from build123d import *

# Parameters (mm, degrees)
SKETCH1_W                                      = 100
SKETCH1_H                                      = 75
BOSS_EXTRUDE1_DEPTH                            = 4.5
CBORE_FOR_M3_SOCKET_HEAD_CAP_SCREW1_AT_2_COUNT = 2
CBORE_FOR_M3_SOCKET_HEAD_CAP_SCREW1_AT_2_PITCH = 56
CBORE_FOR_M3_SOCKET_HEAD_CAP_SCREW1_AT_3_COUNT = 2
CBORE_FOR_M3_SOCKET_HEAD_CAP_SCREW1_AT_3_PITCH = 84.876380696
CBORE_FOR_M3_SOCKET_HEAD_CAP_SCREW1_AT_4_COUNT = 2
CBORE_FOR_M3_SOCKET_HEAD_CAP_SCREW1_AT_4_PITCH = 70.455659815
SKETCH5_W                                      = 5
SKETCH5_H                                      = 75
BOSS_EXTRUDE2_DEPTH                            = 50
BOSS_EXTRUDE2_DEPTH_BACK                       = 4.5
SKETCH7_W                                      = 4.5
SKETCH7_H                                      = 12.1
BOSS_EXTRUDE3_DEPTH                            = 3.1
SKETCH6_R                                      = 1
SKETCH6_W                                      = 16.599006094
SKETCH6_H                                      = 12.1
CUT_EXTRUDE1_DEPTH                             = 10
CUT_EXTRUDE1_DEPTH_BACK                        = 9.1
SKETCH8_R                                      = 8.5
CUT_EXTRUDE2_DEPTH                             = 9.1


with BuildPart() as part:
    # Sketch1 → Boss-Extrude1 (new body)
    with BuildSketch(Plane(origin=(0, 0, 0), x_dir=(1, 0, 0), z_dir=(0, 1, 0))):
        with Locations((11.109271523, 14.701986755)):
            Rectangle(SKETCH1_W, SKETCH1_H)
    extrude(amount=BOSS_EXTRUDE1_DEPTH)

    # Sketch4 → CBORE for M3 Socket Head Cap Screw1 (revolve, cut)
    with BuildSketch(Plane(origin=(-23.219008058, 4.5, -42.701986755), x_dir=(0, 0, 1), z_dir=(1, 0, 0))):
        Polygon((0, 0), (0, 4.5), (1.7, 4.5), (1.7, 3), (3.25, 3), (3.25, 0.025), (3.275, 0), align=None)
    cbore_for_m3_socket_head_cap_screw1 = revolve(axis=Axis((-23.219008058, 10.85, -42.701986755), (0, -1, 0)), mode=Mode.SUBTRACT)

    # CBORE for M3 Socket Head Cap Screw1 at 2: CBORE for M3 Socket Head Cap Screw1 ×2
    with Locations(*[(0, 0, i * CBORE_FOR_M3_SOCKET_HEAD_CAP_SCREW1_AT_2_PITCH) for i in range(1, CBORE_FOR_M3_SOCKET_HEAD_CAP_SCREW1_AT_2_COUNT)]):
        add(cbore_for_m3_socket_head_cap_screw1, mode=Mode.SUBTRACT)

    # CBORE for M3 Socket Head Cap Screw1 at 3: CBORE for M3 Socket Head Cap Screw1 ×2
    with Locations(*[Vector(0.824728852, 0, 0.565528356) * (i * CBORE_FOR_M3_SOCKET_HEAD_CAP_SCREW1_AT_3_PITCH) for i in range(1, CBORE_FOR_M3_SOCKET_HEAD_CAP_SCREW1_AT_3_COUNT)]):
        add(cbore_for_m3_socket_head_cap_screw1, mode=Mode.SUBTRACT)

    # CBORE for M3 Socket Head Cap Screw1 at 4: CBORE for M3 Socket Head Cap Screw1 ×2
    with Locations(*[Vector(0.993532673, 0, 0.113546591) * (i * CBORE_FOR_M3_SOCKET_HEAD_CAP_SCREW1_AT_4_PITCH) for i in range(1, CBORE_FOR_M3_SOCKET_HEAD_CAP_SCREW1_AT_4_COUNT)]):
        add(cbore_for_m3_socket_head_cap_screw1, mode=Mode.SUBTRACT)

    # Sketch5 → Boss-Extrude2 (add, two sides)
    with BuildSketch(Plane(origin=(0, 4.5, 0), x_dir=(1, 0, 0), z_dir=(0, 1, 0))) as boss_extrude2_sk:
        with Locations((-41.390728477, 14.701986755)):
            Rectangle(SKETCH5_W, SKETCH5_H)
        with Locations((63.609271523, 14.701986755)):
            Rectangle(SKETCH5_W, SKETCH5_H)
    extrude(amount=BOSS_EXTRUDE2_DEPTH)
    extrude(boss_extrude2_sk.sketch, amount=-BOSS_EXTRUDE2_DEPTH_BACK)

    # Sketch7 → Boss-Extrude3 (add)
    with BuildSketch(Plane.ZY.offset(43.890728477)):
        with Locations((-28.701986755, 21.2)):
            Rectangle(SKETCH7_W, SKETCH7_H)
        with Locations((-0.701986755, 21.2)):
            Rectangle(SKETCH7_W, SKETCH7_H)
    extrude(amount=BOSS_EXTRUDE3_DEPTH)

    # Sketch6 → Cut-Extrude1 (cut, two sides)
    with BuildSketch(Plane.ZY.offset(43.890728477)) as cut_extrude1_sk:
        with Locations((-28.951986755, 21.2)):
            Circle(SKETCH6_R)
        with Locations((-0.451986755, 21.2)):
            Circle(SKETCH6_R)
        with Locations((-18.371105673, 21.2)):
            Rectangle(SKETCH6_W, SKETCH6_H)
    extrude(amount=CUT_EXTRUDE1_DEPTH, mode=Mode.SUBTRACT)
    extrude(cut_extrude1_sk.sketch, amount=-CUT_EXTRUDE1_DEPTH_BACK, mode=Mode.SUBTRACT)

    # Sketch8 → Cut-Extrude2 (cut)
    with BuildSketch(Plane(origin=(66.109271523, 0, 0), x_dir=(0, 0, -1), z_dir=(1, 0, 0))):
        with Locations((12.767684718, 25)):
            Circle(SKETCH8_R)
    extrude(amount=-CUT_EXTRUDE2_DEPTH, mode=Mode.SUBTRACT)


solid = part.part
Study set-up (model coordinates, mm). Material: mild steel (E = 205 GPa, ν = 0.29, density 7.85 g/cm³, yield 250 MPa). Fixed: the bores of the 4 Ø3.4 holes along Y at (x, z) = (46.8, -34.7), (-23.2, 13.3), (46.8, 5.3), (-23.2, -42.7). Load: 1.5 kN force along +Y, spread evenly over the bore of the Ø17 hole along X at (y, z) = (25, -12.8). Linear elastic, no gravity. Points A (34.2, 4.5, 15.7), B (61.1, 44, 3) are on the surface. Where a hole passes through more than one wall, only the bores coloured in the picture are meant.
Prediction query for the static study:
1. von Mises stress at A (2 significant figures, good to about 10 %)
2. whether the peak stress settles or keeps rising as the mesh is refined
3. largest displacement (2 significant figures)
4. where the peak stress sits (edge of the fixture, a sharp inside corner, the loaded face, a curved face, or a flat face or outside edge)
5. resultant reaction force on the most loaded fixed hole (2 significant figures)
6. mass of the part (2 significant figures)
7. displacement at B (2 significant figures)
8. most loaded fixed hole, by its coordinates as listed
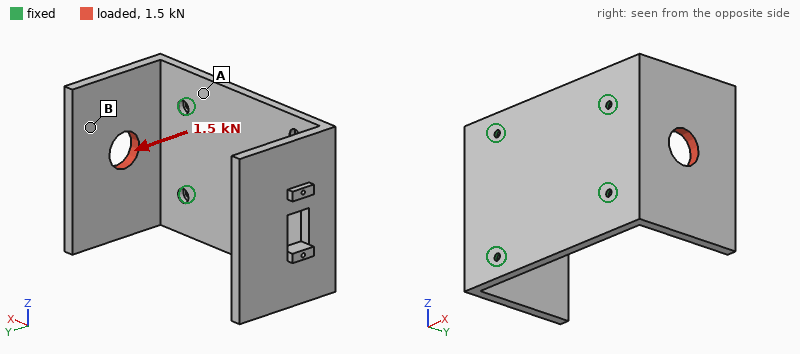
48 MPa
keeps rising
0.23 mm
edge of the fixture
1.5 kN
570 g
0.18 mm
(46.8, 5.3)
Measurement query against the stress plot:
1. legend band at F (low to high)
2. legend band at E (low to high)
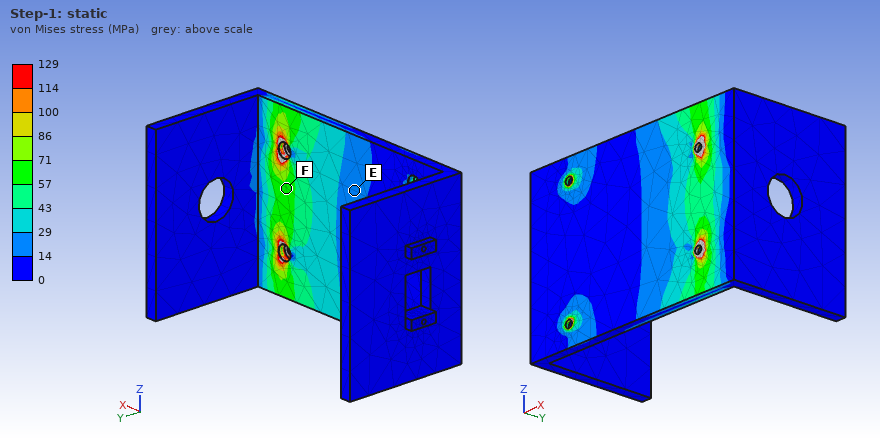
57 to 71 MPa
14 to 29 MPa
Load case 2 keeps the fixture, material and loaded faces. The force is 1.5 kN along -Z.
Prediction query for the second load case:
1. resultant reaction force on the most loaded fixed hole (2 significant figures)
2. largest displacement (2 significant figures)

1.4 kN
81 µm
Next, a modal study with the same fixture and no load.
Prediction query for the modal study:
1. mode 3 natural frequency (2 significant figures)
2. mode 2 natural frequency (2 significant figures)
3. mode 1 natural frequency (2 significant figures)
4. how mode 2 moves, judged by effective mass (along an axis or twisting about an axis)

1700 Hz
750 Hz
700 Hz
along X
